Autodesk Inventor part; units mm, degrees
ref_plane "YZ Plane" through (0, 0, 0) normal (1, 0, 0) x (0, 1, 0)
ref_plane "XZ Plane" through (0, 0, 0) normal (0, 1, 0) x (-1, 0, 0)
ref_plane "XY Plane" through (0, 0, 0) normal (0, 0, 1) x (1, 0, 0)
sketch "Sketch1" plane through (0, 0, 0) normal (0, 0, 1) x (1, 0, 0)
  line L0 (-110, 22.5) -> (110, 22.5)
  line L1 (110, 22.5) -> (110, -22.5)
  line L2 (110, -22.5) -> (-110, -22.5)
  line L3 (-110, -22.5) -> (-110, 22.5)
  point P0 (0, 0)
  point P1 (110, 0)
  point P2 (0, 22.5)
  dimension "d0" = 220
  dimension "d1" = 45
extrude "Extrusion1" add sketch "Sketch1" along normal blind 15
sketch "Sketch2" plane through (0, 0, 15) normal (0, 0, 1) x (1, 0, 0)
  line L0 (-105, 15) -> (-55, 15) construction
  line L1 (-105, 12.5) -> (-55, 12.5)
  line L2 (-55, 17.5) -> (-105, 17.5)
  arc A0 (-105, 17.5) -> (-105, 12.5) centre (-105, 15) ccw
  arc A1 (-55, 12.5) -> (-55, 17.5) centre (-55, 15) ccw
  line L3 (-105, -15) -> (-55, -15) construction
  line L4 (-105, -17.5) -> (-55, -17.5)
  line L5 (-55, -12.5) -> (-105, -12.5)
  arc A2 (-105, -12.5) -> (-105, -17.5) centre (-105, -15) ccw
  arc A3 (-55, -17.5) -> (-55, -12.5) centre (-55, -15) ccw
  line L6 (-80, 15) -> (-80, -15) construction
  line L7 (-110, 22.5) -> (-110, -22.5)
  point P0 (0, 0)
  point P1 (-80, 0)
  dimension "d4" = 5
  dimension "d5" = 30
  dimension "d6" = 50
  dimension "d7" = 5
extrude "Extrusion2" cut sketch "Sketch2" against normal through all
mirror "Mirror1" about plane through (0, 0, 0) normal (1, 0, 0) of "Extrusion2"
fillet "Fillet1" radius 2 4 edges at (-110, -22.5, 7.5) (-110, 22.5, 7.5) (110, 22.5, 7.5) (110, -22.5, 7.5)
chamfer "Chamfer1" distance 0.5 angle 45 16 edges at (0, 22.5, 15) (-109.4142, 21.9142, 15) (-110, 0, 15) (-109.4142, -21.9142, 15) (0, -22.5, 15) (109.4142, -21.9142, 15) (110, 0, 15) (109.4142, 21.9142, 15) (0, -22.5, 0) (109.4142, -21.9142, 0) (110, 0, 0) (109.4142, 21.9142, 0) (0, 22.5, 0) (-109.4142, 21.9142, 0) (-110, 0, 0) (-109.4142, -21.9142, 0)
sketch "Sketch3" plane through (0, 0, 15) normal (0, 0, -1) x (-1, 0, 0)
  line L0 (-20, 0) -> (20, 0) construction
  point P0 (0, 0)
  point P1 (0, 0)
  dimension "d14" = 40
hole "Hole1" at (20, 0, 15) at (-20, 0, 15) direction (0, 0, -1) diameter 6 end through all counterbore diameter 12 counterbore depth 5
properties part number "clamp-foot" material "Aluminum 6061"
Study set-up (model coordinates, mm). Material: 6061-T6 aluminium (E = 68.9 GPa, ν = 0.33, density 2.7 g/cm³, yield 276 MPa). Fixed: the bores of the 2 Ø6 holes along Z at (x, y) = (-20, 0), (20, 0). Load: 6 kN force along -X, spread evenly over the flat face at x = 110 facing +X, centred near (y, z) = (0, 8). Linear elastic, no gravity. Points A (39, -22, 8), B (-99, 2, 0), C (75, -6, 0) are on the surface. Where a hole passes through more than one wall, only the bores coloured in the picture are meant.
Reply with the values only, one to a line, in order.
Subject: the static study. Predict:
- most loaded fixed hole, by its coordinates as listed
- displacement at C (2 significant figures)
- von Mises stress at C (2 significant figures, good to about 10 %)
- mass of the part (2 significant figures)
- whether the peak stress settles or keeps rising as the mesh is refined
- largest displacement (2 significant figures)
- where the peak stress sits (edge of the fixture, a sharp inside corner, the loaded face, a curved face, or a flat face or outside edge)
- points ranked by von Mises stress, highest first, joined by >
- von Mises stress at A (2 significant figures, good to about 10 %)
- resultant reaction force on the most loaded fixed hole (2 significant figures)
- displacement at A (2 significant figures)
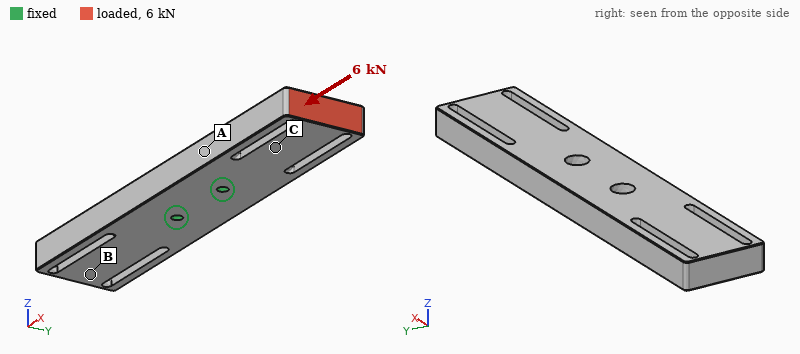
(20, 0)
13 µm
12 MPa
350 g
keeps rising
25 µm
edge of the fixture
C > A > B
6.9 MPa
4.4 kN
5.9 µm
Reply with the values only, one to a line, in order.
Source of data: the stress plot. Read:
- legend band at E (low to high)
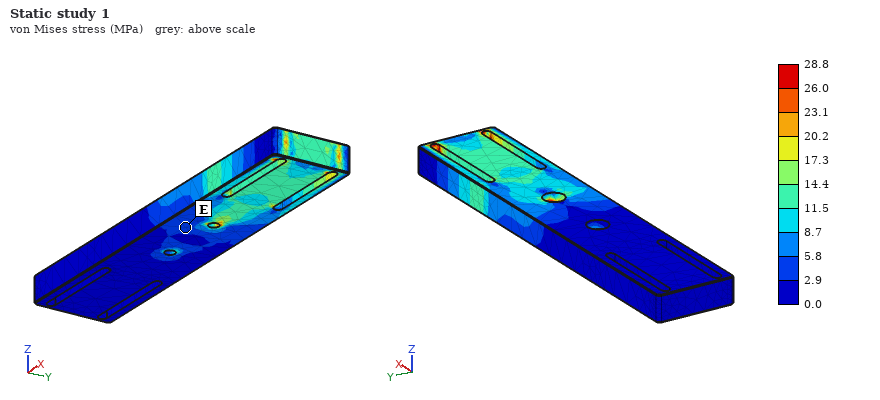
2.9 to 5.8 MPa
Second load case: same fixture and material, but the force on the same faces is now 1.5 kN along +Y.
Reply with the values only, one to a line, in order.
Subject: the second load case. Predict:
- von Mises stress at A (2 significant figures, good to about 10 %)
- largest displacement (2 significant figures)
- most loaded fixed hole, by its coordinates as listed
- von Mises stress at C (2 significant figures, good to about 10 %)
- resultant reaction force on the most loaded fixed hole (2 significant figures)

19 MPa
0.14 mm
(20, 0)
12 MPa
4.4 kN
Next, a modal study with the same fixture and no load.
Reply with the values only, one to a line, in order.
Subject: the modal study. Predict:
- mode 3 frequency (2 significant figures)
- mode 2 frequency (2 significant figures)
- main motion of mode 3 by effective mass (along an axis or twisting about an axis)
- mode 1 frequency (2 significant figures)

2500 Hz
1400 Hz
twisting about Z
1400 Hz
